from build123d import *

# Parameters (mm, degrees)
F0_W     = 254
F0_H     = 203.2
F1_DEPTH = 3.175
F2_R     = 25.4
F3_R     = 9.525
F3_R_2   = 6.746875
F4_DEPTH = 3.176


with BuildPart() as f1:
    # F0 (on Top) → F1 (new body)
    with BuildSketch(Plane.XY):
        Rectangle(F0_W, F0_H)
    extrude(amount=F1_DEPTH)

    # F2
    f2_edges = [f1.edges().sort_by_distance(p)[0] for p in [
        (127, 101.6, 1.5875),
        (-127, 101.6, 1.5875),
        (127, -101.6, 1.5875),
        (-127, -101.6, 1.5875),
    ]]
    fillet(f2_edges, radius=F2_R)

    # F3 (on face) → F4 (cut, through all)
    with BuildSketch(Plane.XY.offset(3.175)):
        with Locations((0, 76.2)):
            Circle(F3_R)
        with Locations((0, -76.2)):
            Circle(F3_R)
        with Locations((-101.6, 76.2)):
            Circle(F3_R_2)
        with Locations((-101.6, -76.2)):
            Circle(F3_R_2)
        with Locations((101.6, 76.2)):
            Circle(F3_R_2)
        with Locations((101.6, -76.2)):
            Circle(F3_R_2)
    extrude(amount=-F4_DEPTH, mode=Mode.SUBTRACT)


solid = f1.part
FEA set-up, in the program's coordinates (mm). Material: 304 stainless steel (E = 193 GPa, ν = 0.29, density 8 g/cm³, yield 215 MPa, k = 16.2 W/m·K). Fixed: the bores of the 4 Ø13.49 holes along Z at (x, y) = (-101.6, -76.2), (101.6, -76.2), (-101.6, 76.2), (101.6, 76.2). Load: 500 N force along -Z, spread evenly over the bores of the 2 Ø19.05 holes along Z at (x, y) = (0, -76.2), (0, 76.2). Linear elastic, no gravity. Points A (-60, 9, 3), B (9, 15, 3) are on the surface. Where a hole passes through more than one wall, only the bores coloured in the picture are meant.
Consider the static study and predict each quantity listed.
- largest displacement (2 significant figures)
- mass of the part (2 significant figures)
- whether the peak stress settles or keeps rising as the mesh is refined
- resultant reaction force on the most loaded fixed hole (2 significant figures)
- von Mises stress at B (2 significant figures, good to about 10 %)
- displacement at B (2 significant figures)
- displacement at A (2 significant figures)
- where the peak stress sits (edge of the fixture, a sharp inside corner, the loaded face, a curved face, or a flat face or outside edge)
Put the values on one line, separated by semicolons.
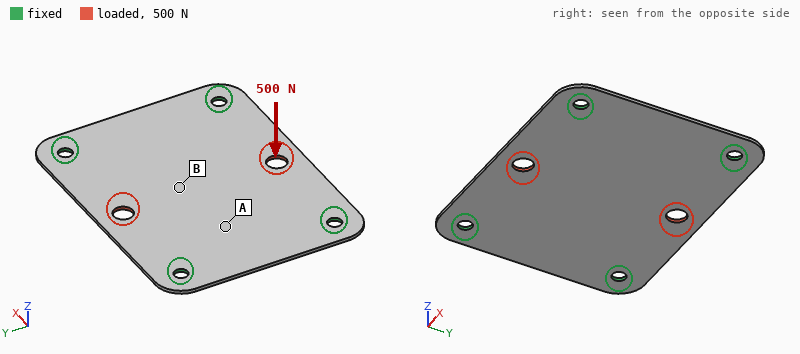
0.31 mm; 1.3 kg; keeps rising; 130 N; 23 MPa; 0.19 mm; 0.093 mm; edge of the fixture
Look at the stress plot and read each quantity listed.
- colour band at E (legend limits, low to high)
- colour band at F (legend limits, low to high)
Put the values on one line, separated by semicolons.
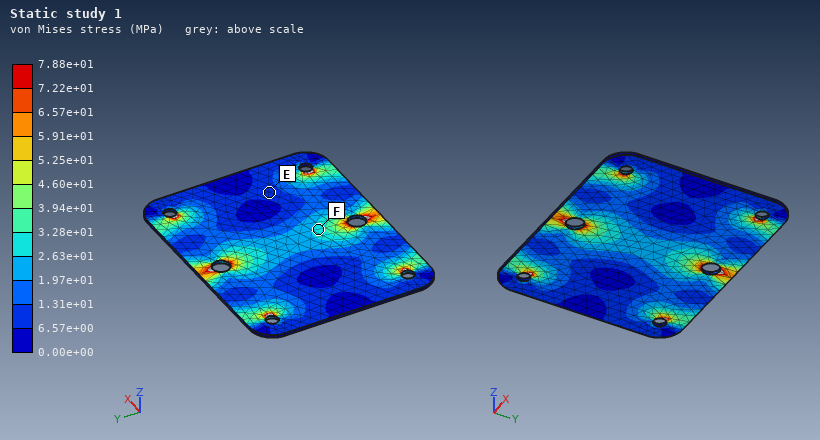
6.57e+00 to 1.31e+01 MPa; 2.63e+01 to 3.28e+01 MPa
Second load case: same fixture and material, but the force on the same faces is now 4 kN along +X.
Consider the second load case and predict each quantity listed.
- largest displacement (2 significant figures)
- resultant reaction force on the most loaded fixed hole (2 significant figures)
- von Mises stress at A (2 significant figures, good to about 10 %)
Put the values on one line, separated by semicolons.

3.5 µm; 1.0 kN; 1.3 MPa
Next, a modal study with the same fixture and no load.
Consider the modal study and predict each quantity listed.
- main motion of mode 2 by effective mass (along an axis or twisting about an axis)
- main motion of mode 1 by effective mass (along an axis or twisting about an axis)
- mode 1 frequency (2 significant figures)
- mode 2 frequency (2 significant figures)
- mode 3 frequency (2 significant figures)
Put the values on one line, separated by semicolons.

twisting about X; along Z; 340 Hz; 490 Hz; 670 Hz
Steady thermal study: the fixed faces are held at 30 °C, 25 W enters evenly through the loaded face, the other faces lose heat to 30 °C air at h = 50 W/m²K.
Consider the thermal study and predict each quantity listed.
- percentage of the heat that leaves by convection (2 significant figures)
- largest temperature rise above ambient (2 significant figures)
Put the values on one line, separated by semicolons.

98 %; 56 K
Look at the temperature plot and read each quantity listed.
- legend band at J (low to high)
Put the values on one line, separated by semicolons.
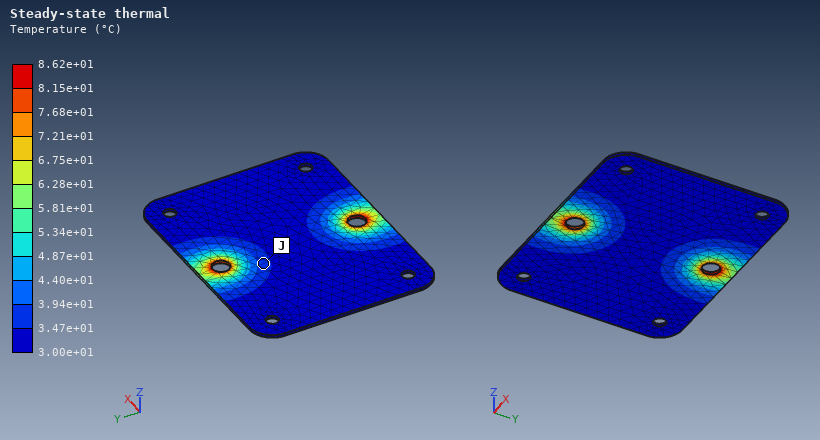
3.47e+01 to 3.94e+01 °C
